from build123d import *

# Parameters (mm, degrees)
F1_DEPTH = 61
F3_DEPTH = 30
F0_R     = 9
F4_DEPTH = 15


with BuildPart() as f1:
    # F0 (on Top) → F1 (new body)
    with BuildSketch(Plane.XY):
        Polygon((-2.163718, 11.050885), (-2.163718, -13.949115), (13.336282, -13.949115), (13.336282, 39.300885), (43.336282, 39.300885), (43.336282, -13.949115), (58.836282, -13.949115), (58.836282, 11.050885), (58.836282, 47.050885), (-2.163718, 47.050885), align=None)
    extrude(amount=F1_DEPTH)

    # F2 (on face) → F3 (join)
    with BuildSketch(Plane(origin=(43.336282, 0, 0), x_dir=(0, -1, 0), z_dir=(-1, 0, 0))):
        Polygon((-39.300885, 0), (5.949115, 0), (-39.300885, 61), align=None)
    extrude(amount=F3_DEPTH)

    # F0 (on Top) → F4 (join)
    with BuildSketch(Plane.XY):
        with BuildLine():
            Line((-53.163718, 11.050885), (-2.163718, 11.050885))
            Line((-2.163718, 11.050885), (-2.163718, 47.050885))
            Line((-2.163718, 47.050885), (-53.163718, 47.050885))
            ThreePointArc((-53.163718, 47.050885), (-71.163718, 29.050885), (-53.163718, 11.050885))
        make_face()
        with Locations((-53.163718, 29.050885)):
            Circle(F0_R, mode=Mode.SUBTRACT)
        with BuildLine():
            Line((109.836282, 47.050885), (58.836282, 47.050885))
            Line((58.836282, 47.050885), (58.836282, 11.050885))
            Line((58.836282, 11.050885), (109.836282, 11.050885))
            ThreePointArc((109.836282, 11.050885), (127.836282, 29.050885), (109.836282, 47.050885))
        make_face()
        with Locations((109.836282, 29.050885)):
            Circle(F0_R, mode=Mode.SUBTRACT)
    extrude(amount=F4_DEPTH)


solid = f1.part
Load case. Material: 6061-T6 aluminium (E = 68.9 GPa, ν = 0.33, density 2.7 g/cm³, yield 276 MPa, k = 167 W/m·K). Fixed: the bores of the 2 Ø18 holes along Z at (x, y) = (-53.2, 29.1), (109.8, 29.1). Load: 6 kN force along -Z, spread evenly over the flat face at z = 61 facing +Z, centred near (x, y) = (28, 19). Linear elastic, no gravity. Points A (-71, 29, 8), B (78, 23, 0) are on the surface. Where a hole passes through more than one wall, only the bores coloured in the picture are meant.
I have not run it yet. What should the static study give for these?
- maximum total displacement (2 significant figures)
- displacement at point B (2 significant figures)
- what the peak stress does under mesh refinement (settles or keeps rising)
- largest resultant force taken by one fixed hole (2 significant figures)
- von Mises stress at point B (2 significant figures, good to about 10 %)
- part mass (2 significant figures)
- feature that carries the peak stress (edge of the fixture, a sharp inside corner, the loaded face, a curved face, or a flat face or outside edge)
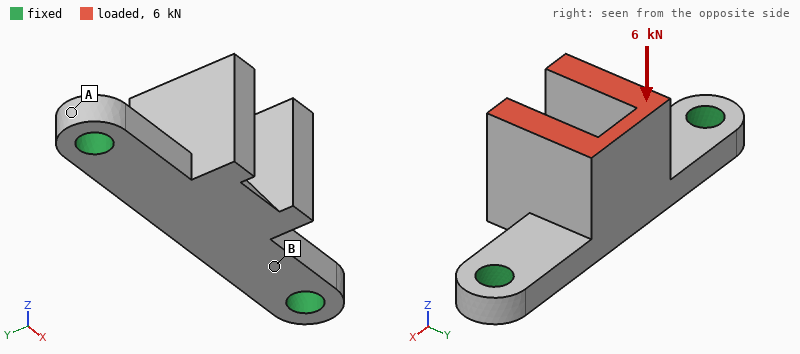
0.16 mm
0.039 mm
keeps rising
3.3 kN
22 MPa
630 g
edge of the fixture
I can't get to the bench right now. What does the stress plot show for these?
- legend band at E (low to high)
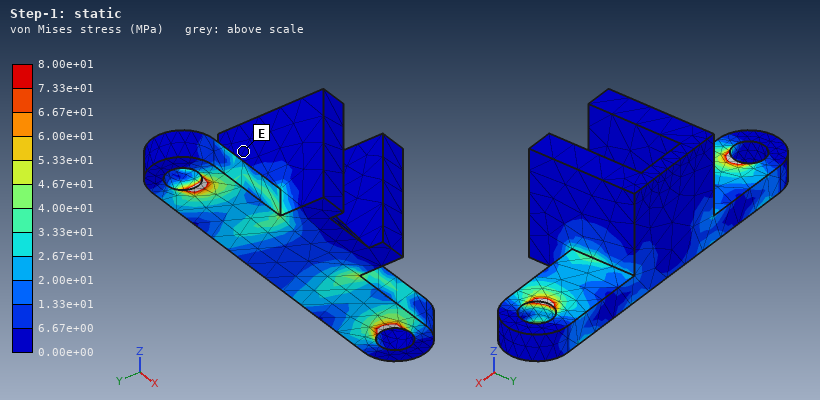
0.00e+00 to 6.67e+00 MPa
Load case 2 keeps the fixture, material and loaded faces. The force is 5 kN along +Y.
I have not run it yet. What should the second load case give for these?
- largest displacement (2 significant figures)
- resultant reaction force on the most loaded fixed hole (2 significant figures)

0.55 mm
2.5 kN
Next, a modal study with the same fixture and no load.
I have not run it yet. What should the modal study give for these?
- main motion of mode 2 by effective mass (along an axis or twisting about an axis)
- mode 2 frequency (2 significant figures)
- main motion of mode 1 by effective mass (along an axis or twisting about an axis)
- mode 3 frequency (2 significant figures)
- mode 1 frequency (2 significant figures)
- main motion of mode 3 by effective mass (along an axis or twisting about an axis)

along Z
2300 Hz
along Y
3400 Hz
1300 Hz
along X
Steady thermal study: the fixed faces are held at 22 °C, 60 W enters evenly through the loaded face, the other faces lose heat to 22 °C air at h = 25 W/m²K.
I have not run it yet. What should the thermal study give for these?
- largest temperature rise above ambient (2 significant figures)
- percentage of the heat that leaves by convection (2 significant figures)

22 K
18 %
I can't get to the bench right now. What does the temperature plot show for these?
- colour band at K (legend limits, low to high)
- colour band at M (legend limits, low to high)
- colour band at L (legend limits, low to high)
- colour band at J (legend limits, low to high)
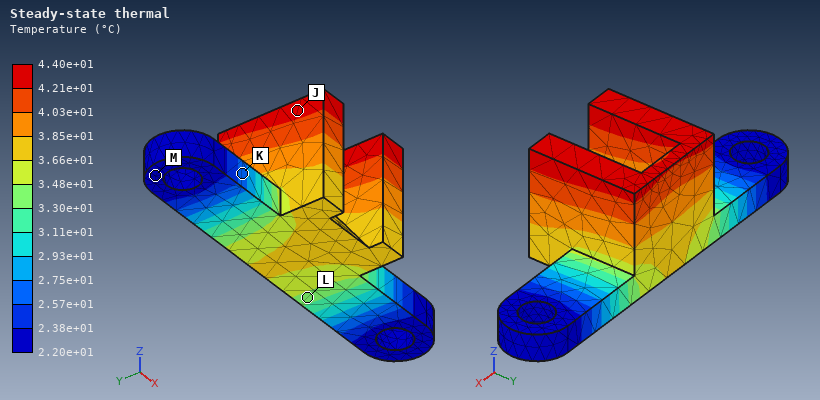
2.57e+01 to 2.75e+01 °C
2.20e+01 to 2.38e+01 °C
3.30e+01 to 3.48e+01 °C
4.21e+01 to 4.40e+01 °C
